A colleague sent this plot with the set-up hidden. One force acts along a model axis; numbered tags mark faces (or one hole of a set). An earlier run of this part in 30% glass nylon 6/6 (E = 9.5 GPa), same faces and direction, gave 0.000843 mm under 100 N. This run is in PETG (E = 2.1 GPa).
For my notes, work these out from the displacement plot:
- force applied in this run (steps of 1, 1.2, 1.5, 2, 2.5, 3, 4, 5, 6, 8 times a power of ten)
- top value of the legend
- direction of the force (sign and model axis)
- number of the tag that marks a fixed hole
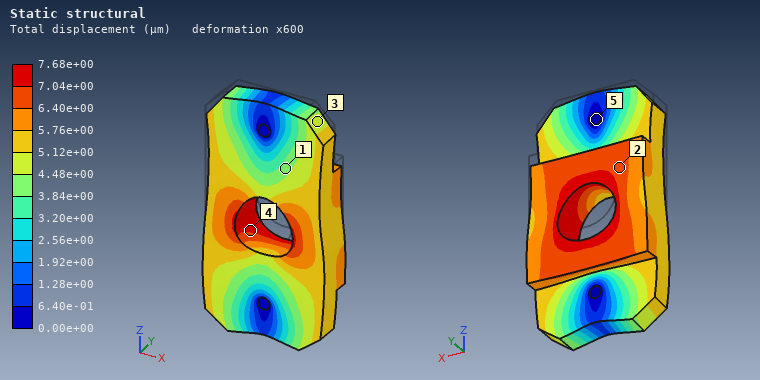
200 N
7.68e+00 µm
-Z
5
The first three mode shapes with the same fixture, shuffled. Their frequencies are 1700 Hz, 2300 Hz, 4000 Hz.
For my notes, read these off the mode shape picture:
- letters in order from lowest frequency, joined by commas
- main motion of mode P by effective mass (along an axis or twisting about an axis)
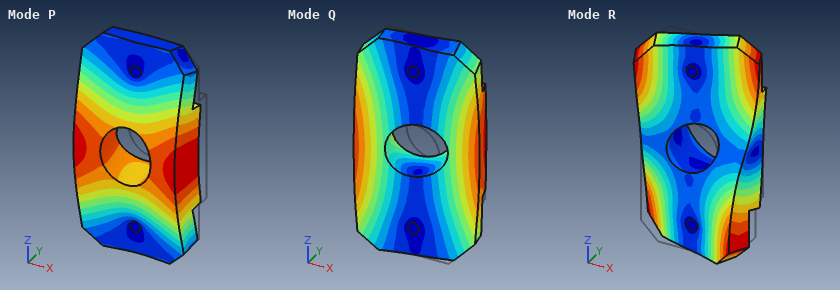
Q, P, R
along Y
